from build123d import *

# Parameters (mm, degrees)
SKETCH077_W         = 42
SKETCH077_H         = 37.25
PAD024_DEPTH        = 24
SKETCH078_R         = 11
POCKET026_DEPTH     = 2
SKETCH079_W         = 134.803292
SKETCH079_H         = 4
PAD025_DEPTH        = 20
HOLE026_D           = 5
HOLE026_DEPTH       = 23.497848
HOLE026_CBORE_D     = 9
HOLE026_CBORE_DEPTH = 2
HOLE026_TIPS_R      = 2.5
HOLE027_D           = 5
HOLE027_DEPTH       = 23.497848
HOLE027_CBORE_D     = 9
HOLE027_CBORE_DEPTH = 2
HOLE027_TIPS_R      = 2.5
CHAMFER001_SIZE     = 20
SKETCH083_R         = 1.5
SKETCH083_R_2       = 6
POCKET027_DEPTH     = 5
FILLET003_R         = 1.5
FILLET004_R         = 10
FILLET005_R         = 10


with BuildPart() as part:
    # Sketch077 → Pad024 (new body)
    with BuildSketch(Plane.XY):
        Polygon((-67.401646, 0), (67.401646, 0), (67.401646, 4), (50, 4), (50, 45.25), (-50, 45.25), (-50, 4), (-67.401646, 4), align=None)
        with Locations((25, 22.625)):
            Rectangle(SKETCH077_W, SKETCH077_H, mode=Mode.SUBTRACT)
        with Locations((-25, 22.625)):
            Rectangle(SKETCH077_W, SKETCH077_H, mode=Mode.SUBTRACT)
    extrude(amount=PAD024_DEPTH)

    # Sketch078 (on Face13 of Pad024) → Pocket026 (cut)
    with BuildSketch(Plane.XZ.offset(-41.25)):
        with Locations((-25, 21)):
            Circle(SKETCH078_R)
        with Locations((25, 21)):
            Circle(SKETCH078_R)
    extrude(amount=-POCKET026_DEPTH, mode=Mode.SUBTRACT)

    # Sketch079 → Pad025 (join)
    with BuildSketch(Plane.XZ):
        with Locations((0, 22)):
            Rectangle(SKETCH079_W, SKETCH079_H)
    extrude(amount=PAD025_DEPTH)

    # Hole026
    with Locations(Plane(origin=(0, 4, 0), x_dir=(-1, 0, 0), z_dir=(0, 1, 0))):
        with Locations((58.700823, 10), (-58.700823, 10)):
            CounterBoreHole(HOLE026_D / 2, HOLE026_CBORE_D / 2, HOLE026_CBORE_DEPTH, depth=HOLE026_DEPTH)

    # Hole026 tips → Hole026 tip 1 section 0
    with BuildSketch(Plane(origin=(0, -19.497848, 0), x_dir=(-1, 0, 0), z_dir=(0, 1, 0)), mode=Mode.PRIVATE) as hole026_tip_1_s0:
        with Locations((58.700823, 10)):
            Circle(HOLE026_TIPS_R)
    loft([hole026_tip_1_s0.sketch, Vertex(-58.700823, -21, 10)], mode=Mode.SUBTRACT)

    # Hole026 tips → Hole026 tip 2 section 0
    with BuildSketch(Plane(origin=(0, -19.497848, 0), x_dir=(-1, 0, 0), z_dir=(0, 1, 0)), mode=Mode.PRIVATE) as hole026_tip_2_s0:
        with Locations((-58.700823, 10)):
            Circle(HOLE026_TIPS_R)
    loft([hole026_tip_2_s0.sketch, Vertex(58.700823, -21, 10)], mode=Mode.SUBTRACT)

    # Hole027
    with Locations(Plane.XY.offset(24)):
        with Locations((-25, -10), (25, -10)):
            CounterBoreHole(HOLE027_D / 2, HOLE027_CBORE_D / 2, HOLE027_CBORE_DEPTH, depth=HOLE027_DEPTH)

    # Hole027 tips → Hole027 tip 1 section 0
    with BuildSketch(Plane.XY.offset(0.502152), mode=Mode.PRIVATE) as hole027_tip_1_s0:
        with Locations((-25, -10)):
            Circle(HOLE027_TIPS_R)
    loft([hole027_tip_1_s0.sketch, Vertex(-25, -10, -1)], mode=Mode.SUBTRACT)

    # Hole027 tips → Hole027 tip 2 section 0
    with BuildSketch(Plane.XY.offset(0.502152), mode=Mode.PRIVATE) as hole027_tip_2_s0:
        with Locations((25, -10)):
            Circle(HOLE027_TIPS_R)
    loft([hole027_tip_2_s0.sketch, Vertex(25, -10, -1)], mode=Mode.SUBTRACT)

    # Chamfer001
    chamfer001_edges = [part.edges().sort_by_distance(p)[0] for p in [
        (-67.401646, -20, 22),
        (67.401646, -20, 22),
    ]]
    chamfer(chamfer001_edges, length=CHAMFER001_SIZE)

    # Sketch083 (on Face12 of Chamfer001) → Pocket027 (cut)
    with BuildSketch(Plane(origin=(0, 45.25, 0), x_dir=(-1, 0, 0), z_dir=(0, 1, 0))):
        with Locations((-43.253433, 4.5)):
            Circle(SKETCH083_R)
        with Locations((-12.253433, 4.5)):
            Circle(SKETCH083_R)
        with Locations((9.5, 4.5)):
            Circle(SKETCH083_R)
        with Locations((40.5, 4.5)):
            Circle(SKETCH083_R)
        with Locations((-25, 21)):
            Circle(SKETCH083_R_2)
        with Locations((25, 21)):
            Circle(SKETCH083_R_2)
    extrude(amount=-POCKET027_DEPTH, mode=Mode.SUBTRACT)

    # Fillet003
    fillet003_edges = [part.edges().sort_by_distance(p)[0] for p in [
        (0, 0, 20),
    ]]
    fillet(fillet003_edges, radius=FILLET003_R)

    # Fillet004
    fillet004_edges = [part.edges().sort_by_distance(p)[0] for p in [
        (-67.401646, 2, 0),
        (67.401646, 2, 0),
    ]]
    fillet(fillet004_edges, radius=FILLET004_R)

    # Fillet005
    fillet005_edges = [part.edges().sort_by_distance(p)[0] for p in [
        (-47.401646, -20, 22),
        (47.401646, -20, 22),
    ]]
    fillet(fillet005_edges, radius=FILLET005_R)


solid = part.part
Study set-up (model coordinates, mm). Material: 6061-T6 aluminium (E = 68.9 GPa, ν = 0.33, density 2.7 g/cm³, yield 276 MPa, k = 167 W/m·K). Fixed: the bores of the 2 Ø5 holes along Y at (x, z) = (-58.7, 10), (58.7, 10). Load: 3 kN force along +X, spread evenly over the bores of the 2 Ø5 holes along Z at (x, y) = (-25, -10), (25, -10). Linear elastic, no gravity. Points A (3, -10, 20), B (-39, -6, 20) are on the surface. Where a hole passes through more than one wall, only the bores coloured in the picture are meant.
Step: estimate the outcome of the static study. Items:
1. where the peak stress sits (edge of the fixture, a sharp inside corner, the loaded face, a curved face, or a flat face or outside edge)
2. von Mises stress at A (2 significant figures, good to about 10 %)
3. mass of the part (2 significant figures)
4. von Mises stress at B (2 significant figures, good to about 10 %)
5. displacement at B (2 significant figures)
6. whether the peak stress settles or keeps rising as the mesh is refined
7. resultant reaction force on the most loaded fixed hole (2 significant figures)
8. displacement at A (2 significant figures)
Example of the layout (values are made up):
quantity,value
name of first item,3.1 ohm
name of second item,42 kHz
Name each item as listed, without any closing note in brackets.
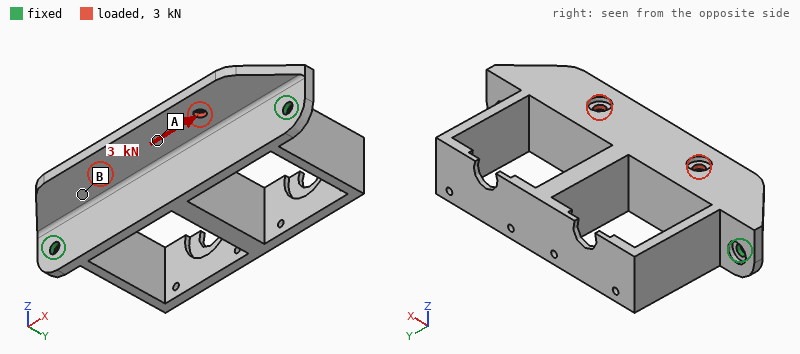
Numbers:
quantity,value
where the peak stress sits,edge of the fixture
von Mises stress at A,9.5 MPa
mass of the part,120 g
von Mises stress at B,20 MPa
displacement at B,23 µm
whether the peak stress settles or keeps rising as the mesh is refined,keeps rising
resultant reaction force on the most loaded fixed hole,1.5 kN
displacement at A,18 µm
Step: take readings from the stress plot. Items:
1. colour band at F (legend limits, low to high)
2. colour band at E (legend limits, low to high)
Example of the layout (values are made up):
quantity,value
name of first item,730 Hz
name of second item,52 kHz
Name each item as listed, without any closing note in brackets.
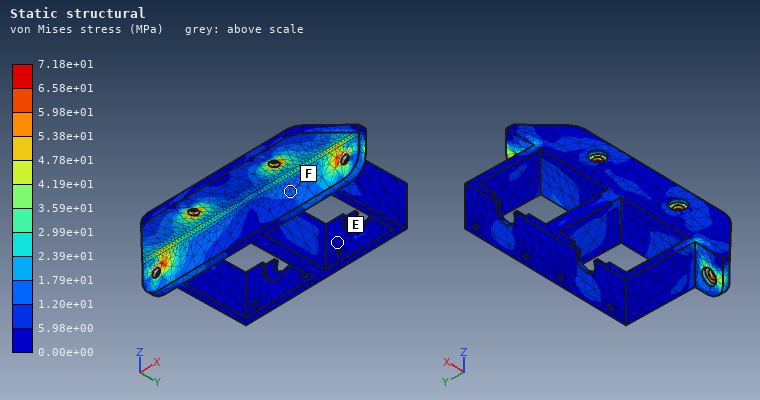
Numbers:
quantity,value
colour band at F,1.20e+01 to 1.79e+01 MPa
colour band at E,0.00e+00 to 5.98e+00 MPa
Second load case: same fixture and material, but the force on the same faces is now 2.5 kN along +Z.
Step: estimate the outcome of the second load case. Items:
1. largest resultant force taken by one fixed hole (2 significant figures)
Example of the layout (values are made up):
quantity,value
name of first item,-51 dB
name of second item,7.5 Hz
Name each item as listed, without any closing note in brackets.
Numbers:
quantity,value
largest resultant force taken by one fixed hole,1.4 kN
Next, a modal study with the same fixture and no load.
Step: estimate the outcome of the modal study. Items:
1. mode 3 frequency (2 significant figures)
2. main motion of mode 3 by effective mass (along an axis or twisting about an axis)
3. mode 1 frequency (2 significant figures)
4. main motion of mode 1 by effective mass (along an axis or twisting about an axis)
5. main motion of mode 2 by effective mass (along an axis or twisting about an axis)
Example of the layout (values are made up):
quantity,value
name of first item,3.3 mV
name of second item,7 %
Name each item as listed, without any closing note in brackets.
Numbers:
quantity,value
mode 3 frequency,2200 Hz
main motion of mode 3 by effective mass,along Y
mode 1 frequency,790 Hz
main motion of mode 1 by effective mass,along Z
main motion of mode 2 by effective mass,along X
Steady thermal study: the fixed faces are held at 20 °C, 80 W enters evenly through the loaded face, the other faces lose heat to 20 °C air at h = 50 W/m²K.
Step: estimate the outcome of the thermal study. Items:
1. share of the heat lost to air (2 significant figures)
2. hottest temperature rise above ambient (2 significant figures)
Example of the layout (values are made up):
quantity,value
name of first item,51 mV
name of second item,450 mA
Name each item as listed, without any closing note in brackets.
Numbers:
quantity,value
share of the heat lost to air,41 %
hottest temperature rise above ambient,72 K
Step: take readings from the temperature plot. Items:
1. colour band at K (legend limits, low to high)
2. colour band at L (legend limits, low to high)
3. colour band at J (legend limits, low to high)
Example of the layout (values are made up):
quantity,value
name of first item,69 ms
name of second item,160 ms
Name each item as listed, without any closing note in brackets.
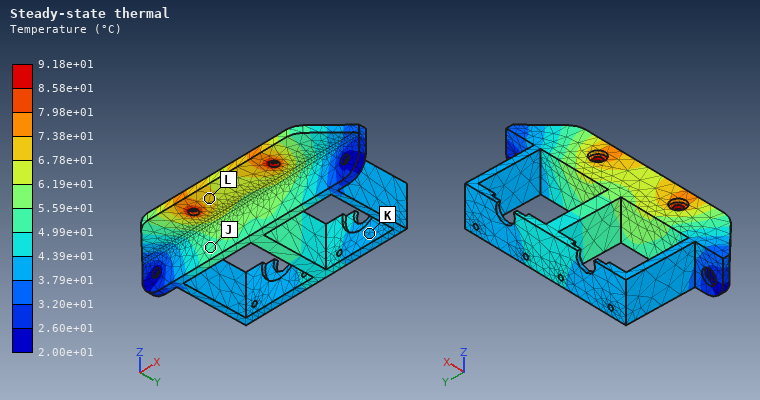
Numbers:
quantity,value
colour band at K,3.79e+01 to 4.39e+01 °C
colour band at L,6.78e+01 to 7.38e+01 °C
colour band at J,4.99e+01 to 5.59e+01 °C
